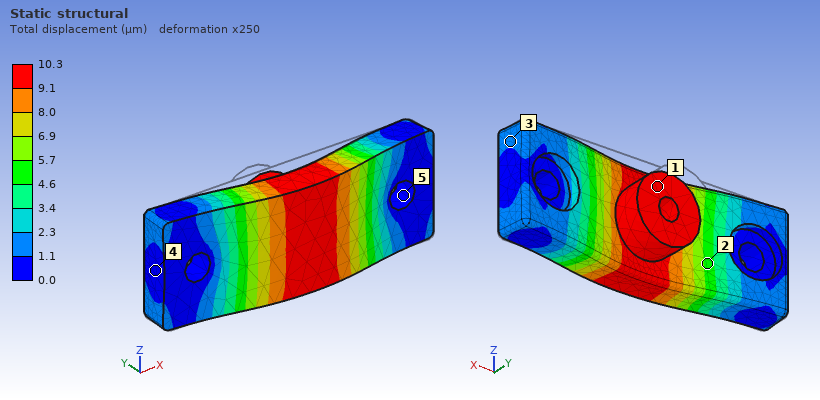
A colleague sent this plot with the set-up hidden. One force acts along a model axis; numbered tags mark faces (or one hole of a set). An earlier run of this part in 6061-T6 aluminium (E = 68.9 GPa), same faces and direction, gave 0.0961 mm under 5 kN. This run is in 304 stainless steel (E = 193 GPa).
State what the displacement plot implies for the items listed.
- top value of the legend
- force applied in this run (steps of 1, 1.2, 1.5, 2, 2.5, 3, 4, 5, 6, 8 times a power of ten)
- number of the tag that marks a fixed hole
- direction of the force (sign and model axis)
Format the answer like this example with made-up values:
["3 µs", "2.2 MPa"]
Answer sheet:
["10.3 µm", "1.5 kN", "5", "-Y"]
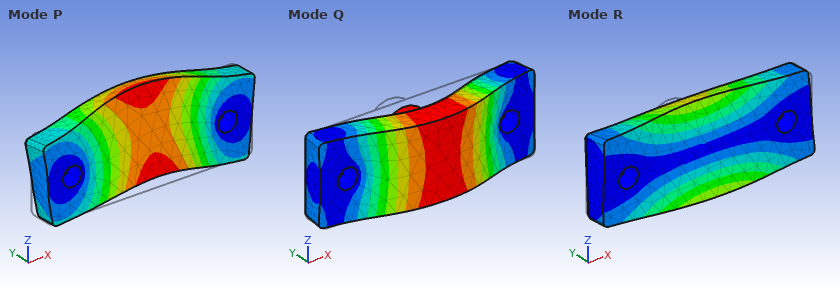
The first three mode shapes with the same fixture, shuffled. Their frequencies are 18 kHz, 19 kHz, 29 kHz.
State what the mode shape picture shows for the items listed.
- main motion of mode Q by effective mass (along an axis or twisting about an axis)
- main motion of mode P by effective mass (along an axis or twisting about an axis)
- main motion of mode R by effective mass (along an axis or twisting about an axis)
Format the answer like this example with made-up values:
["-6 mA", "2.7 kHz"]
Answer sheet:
["along Y", "along Z", "along Z"]
